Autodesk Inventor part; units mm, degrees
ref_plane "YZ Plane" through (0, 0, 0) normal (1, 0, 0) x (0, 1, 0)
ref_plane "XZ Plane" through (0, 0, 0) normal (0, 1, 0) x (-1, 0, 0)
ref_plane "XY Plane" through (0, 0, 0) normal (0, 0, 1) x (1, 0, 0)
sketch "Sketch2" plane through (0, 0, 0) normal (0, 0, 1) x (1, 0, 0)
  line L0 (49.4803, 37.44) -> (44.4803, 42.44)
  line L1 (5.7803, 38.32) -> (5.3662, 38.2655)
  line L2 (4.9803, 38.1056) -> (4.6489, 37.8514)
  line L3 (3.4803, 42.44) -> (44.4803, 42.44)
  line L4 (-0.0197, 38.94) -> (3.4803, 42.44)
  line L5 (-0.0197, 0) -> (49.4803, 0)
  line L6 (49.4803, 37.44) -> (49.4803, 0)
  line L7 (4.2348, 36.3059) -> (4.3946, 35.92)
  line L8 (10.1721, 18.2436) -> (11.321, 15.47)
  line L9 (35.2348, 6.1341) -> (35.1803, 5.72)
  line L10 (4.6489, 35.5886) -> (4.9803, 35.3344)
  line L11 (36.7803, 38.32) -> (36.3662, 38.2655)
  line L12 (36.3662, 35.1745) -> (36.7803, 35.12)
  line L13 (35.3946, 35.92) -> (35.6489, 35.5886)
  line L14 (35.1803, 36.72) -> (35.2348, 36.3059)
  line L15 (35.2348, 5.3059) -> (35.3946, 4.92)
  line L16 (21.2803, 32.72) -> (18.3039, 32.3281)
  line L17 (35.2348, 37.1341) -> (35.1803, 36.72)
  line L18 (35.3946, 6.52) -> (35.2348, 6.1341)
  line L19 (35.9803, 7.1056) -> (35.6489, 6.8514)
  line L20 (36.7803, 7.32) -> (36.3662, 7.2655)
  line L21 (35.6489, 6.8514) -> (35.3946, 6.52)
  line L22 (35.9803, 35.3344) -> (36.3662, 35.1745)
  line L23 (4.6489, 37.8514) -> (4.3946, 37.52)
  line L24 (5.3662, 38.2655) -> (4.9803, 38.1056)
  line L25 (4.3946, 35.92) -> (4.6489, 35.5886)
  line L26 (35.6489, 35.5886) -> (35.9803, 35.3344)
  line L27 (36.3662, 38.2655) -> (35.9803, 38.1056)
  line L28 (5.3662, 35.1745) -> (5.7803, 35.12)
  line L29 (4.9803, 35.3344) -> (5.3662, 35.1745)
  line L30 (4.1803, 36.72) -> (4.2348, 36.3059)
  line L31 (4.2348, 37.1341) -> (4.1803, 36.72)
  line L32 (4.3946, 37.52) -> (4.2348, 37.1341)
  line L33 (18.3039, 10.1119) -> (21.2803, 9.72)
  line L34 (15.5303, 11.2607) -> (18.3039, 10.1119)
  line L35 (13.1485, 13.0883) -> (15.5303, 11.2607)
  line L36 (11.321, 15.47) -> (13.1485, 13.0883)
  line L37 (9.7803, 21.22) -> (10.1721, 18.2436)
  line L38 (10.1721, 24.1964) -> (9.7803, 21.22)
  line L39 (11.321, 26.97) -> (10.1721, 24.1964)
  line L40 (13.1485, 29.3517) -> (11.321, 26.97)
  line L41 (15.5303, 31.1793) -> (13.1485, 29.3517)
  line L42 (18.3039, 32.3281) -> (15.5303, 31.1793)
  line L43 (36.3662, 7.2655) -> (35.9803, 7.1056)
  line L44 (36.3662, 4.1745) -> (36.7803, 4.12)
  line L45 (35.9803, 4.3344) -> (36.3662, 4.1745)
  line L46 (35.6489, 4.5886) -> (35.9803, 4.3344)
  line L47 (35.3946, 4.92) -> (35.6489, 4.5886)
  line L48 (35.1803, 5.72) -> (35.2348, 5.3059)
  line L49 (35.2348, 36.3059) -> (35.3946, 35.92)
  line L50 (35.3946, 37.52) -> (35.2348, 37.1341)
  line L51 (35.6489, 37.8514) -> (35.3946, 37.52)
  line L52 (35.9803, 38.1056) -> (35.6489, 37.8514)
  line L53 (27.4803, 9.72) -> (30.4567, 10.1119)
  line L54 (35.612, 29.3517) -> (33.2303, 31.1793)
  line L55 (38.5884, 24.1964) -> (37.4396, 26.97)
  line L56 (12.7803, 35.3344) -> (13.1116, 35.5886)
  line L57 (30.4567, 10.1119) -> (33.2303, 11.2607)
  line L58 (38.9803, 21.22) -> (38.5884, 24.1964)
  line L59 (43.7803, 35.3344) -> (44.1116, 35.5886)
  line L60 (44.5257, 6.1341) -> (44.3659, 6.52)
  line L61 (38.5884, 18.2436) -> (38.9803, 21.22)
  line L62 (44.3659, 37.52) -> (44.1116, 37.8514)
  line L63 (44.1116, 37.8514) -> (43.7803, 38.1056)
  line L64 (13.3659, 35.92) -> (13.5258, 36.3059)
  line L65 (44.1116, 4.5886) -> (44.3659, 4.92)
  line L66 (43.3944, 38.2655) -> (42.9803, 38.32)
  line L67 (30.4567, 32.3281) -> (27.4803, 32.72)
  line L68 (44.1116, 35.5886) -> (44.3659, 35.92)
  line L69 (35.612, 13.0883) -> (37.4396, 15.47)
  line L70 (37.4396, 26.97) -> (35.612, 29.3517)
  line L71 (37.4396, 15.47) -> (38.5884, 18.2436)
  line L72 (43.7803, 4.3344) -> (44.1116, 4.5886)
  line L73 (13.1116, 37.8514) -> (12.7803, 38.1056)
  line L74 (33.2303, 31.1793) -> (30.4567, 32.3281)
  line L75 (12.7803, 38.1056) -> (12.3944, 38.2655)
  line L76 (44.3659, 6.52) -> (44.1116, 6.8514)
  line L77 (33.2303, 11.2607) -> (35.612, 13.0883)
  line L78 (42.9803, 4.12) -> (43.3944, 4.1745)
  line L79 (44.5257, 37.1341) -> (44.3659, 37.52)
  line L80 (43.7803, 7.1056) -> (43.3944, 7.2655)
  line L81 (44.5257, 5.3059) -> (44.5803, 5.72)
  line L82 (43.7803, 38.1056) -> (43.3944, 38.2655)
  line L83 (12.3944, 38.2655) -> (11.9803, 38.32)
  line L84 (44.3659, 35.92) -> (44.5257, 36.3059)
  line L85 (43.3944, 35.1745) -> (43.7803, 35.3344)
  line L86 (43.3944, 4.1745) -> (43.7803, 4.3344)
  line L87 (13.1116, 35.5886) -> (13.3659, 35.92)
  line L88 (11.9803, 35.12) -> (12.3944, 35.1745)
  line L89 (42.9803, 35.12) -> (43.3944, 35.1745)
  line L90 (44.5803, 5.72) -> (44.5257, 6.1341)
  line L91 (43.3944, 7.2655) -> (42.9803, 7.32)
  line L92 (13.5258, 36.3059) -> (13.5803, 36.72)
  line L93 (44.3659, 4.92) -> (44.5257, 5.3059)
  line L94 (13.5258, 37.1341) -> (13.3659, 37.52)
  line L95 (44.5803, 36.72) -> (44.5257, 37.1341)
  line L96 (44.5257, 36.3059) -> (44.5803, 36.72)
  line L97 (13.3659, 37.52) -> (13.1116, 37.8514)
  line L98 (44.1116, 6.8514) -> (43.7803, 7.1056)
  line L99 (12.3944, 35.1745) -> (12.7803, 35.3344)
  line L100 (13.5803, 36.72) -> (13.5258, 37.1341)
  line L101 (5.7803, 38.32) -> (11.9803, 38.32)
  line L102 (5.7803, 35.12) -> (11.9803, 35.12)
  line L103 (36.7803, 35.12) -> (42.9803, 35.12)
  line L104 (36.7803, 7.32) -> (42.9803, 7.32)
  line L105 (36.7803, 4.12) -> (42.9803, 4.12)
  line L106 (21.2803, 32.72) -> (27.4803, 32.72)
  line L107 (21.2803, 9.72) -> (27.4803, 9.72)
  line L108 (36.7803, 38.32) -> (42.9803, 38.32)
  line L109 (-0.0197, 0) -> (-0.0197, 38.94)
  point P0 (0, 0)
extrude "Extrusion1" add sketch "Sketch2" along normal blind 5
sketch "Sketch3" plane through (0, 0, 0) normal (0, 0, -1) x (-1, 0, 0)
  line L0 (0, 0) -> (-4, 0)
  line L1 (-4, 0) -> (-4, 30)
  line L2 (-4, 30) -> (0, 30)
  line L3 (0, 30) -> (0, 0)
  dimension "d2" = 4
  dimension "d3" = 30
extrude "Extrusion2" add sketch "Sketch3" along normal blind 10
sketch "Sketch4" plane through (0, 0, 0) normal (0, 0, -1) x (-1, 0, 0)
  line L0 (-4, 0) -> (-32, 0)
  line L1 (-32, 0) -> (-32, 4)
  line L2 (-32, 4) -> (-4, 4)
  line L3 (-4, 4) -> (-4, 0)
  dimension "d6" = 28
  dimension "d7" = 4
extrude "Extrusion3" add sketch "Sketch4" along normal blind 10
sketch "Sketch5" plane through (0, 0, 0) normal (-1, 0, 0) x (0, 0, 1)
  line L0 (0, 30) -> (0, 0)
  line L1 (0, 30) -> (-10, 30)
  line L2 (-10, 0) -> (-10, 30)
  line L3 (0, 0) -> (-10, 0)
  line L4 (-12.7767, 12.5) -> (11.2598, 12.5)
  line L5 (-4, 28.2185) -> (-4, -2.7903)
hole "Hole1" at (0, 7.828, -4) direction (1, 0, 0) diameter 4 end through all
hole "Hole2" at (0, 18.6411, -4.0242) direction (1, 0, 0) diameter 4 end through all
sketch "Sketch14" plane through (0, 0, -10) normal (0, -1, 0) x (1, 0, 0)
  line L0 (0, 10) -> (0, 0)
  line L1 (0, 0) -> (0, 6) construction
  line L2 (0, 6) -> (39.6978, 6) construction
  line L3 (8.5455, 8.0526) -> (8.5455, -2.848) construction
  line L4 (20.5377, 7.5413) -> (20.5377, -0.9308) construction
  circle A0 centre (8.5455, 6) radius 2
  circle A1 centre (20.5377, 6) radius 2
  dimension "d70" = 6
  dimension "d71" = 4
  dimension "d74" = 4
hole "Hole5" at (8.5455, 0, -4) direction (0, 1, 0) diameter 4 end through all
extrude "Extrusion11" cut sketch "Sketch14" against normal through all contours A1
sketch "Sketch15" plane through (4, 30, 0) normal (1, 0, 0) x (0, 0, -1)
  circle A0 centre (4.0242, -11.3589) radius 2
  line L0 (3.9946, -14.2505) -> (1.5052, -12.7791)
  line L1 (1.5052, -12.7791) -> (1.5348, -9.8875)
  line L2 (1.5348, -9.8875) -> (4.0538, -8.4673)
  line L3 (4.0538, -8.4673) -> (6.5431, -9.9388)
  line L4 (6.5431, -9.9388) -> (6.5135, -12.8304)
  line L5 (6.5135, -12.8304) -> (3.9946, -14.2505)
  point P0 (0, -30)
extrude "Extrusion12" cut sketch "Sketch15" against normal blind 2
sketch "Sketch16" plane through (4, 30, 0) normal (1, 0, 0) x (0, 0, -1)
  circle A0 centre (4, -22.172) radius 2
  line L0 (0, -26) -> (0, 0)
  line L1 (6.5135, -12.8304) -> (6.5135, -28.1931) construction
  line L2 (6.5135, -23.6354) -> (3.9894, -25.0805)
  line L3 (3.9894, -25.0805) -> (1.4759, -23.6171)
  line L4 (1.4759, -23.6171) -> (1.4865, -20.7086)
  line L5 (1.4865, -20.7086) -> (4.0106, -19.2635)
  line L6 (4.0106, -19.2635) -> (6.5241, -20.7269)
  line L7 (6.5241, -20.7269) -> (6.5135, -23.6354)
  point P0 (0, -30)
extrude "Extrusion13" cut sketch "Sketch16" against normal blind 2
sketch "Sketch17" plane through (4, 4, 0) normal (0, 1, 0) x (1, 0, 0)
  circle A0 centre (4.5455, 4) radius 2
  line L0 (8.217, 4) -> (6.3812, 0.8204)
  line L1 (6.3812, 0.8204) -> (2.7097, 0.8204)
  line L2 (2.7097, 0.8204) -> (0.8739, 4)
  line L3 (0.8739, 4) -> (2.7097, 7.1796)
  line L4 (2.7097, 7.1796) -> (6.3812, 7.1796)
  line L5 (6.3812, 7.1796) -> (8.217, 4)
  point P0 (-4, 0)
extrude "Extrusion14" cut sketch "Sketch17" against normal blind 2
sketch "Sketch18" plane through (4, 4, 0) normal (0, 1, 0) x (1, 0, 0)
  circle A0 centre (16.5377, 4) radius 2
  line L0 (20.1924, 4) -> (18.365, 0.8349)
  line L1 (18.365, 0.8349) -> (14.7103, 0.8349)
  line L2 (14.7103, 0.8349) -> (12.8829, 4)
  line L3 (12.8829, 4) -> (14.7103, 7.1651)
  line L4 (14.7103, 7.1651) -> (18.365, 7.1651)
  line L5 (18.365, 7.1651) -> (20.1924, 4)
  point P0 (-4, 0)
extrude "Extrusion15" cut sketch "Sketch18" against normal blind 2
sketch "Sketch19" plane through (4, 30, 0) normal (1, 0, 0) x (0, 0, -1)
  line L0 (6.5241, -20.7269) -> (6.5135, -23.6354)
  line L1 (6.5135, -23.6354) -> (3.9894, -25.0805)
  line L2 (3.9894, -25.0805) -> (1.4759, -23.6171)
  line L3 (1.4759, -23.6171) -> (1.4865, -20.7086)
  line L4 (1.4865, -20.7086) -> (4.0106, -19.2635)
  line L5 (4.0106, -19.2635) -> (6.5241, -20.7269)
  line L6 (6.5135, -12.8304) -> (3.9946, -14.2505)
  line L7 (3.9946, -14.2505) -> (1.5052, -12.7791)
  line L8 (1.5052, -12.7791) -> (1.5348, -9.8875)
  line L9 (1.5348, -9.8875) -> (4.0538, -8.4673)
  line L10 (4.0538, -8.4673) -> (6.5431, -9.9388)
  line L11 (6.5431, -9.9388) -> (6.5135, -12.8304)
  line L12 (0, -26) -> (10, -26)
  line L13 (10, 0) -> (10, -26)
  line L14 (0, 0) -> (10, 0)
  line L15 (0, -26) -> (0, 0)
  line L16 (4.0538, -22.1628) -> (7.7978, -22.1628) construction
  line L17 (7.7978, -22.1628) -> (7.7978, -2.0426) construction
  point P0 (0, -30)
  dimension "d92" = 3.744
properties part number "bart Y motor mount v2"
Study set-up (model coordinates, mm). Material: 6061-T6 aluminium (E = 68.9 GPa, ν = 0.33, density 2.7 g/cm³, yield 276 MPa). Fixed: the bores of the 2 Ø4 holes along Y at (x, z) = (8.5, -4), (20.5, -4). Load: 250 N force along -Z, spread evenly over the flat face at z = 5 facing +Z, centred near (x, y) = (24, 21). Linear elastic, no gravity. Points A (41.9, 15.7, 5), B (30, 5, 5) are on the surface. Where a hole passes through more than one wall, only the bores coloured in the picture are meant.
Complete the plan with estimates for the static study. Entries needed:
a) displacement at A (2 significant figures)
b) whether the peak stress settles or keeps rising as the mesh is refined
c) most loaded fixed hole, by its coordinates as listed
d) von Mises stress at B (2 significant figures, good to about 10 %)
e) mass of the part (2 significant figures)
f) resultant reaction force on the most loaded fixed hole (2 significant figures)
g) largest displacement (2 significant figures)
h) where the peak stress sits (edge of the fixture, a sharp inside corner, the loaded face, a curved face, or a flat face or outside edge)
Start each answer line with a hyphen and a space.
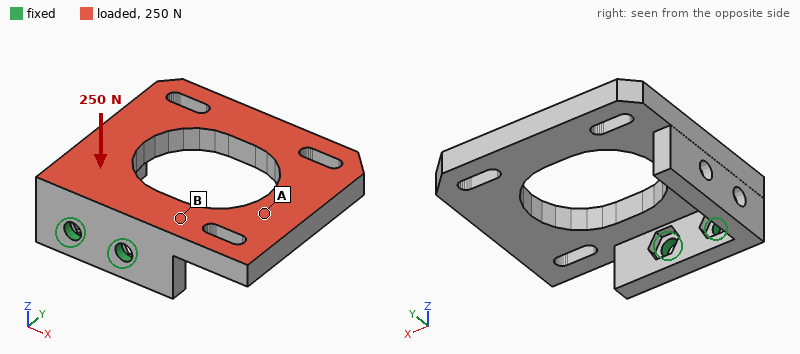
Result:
- 0.10 mm
- keeps rising
- (20.5, -4)
- 34 MPa
- 25 g
- 310 N
- 0.28 mm
- edge of the fixture
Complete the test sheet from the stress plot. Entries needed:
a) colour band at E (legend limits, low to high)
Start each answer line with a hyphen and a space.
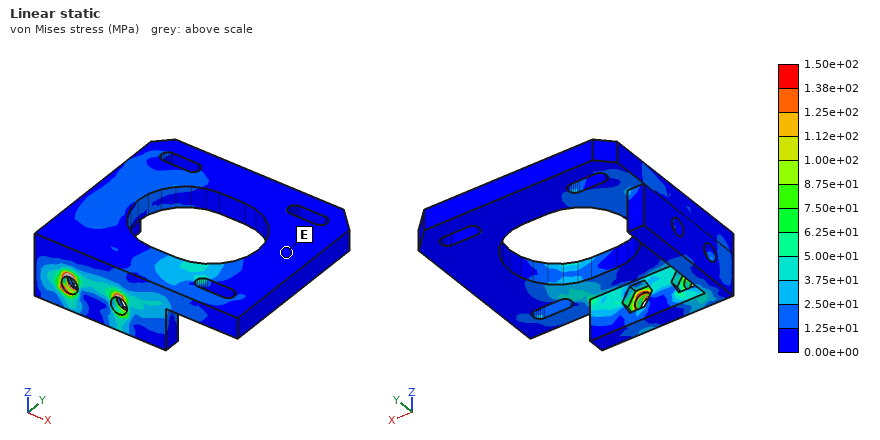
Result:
- 0.00e+00 to 1.25e+01 MPa
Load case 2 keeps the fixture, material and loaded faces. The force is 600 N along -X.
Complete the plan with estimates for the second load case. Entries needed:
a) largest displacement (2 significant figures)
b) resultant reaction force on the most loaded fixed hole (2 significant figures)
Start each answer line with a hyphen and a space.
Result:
- 0.12 mm
- 950 N
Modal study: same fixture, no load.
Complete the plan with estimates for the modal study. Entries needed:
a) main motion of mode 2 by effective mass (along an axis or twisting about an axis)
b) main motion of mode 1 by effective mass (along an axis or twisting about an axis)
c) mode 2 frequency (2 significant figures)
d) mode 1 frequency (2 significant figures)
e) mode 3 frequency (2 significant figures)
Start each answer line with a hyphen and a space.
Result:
- along X
- along Z
- 2400 Hz
- 1400 Hz
- 3400 Hz
